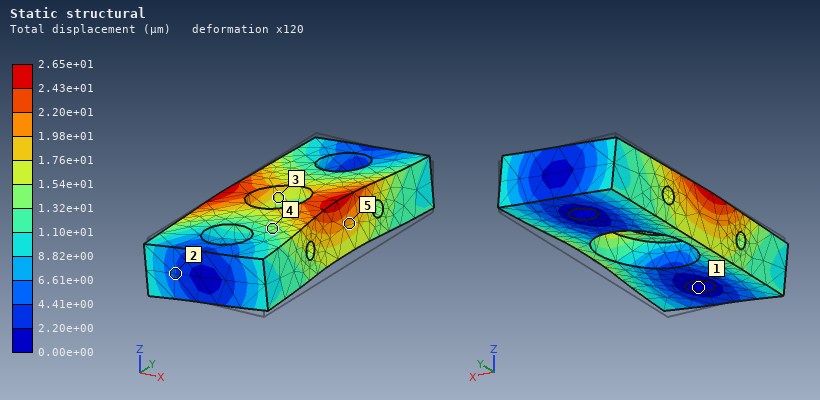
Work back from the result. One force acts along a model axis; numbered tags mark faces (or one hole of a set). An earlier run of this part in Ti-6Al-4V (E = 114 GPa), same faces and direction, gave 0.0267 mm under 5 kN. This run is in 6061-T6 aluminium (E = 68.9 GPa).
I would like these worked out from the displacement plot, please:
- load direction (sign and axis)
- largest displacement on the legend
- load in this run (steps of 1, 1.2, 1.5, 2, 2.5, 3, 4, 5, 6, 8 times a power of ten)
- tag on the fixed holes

-X
2.65e+01 µm
3 kN
1
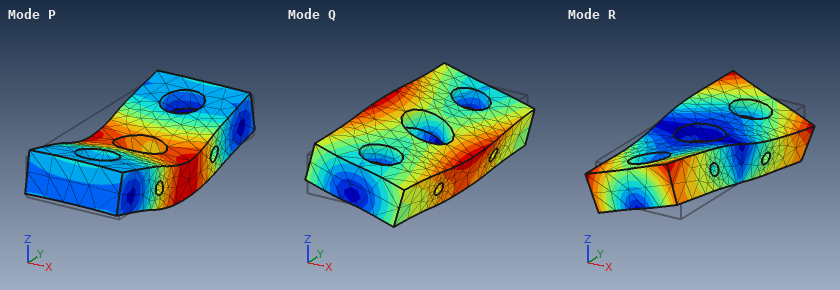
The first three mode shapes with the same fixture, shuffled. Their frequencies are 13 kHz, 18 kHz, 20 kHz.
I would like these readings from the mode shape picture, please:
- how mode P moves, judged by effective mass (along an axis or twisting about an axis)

along Z
